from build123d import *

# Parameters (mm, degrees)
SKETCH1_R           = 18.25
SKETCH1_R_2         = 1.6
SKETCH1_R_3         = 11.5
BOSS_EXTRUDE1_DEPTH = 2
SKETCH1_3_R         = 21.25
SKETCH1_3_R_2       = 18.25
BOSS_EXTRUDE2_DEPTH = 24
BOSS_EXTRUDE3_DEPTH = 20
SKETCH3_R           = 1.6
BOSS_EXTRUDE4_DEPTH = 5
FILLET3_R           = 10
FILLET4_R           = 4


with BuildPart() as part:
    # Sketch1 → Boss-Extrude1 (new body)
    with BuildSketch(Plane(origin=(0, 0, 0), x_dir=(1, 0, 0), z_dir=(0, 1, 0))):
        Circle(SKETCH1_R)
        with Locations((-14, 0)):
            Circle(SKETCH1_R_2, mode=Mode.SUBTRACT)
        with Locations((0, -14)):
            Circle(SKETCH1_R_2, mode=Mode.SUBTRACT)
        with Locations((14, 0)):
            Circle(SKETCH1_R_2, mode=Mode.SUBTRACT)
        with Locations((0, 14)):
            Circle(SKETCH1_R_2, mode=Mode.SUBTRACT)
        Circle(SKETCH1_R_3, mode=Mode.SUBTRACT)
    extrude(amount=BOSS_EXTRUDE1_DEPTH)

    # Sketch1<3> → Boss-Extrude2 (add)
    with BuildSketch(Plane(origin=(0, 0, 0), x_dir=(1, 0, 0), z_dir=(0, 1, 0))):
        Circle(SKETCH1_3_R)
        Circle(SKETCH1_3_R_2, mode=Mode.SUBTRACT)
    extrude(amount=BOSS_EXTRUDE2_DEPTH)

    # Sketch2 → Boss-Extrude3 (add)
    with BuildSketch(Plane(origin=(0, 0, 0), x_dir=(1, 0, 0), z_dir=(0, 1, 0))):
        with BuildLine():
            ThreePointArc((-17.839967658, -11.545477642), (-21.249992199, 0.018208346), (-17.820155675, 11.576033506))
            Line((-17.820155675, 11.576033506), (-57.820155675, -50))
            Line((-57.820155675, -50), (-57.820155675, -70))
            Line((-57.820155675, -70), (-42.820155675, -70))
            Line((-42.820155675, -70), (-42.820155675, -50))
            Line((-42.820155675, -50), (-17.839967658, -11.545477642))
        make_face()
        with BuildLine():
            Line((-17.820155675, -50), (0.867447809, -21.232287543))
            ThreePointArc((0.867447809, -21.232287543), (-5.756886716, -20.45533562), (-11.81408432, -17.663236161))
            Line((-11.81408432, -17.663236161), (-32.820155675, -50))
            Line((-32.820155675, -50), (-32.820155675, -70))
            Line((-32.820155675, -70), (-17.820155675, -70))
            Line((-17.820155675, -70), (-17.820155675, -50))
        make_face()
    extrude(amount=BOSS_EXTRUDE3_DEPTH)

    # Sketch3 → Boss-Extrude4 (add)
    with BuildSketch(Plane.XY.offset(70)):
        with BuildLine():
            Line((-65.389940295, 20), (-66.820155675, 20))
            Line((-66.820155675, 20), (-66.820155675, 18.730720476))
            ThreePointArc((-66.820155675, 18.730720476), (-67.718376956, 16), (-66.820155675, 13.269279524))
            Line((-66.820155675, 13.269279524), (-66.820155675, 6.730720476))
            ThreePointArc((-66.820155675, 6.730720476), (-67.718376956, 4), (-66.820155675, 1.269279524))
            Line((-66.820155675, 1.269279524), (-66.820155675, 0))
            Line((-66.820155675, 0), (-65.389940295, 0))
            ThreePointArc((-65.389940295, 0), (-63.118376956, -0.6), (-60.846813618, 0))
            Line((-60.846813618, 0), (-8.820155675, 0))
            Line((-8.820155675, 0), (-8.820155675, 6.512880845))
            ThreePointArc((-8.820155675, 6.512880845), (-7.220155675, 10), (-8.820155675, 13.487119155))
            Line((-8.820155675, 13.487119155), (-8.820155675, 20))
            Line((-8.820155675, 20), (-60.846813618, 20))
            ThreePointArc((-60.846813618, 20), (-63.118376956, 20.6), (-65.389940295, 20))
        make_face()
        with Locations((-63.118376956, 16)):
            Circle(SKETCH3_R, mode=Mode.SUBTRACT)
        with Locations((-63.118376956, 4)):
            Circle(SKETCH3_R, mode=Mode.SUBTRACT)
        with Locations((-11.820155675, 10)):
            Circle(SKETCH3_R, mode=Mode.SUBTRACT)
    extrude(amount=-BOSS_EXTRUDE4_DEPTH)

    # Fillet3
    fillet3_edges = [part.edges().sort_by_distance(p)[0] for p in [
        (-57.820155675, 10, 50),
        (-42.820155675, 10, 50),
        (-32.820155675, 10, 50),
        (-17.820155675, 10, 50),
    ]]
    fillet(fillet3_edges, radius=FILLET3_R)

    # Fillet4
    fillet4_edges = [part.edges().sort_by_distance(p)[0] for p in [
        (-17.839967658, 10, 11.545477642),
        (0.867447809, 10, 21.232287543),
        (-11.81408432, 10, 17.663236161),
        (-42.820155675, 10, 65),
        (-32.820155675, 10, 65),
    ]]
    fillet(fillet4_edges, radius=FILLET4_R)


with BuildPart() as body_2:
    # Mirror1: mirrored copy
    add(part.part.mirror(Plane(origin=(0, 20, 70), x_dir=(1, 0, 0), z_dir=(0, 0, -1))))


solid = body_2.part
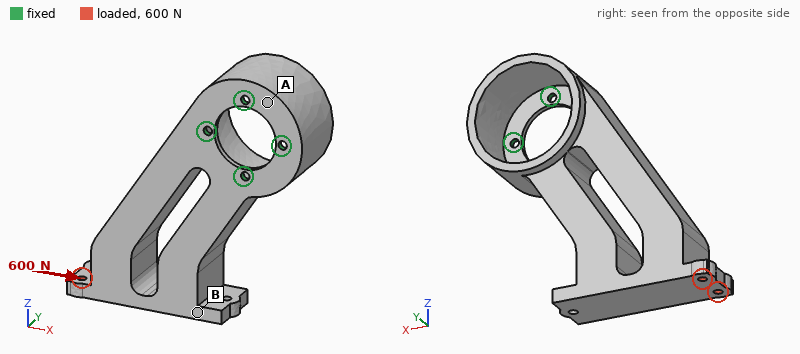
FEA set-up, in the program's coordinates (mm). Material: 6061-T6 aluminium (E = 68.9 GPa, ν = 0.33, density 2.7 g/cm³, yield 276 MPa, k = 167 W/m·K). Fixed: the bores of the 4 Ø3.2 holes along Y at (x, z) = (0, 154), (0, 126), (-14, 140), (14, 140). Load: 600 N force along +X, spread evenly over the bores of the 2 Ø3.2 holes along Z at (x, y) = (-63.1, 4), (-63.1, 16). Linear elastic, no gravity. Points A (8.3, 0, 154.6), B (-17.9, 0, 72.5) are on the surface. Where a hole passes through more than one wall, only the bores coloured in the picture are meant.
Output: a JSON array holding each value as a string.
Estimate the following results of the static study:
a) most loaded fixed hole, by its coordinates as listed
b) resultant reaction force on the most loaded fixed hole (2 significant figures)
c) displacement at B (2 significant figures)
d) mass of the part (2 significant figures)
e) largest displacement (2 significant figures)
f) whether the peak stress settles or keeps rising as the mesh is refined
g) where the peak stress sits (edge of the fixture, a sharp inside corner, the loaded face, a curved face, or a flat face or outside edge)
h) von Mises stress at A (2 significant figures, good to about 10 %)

["(0, 126)", "1.2 kN", "0.090 mm", "130 g", "0.12 mm", "keeps rising", "edge of the fixture", "11 MPa"]
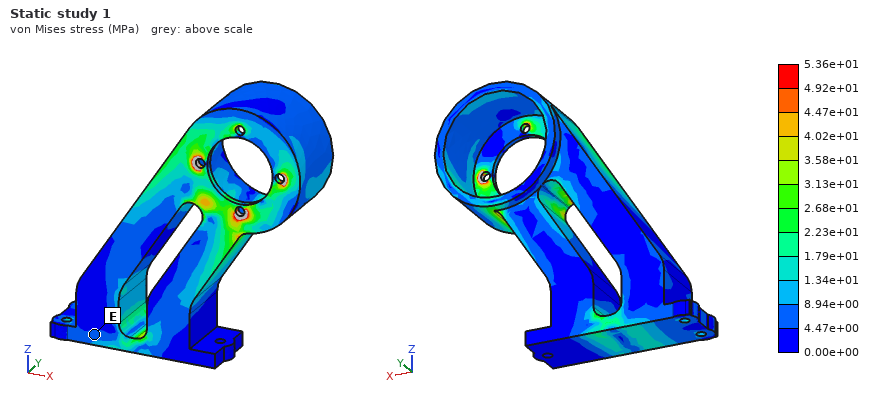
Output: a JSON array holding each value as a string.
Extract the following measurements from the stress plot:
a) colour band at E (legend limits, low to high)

["4.47e+00 to 8.94e+00 MPa"]
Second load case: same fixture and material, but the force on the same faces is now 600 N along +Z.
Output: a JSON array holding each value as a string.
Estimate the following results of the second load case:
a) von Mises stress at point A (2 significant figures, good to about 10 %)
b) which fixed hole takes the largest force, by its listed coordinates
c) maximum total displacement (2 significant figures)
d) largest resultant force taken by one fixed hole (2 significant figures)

["14 MPa", "(-14, 140)", "0.11 mm", "1.1 kN"]
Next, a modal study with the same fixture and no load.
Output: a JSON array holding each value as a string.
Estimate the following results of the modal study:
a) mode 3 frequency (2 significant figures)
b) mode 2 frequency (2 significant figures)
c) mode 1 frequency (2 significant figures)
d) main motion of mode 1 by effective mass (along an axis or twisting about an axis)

["2900 Hz", "1800 Hz", "890 Hz", "along Y"]
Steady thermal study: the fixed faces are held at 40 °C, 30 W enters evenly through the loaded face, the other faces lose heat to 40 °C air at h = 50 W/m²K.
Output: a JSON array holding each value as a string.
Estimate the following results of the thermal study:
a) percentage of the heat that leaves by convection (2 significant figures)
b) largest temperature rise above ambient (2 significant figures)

["41 %", "51 K"]
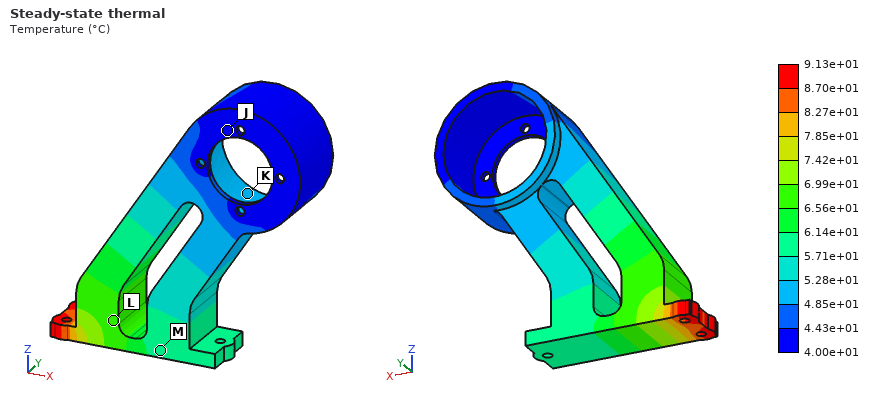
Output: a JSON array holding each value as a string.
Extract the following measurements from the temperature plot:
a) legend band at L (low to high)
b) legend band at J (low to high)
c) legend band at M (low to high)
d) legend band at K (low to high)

["6.56e+01 to 6.99e+01 °C", "4.00e+01 to 4.43e+01 °C", "5.71e+01 to 6.14e+01 °C", "4.85e+01 to 5.28e+01 °C"]
